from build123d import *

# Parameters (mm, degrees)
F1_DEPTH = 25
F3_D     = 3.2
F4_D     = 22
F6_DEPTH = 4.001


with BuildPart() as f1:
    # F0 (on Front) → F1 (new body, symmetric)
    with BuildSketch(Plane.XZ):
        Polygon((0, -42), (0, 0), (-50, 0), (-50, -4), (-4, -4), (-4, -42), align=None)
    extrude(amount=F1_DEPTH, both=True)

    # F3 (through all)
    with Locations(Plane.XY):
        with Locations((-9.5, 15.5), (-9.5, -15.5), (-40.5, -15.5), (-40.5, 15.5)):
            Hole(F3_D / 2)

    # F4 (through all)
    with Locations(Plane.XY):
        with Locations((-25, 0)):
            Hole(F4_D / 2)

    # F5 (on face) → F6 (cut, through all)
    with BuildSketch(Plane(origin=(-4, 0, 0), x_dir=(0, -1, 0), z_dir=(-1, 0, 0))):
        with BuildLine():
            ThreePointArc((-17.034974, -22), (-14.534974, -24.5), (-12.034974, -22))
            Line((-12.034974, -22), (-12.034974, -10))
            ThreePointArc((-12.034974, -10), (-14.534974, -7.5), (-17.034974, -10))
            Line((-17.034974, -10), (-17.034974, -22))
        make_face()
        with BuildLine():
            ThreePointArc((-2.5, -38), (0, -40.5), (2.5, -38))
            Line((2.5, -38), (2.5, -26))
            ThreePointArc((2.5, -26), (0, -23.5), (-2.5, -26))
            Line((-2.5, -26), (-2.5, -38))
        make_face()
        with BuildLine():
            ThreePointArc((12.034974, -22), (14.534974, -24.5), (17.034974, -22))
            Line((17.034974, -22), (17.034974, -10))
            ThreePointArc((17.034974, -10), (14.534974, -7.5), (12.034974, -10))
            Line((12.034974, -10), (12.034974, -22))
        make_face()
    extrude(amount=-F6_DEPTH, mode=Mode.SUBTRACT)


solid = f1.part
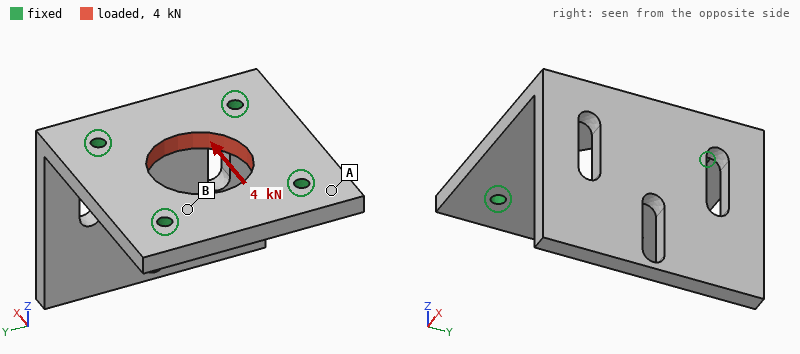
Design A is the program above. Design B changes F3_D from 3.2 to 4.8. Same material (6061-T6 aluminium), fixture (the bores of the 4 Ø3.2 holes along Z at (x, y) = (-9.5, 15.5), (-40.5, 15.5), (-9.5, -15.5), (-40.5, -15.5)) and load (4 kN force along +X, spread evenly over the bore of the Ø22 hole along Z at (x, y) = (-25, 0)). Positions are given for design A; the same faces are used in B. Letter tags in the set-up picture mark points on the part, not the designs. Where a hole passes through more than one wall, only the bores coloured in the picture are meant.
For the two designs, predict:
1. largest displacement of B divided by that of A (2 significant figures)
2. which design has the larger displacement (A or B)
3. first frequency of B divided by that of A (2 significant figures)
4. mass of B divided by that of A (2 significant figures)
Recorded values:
0.89
A
1.0
0.99
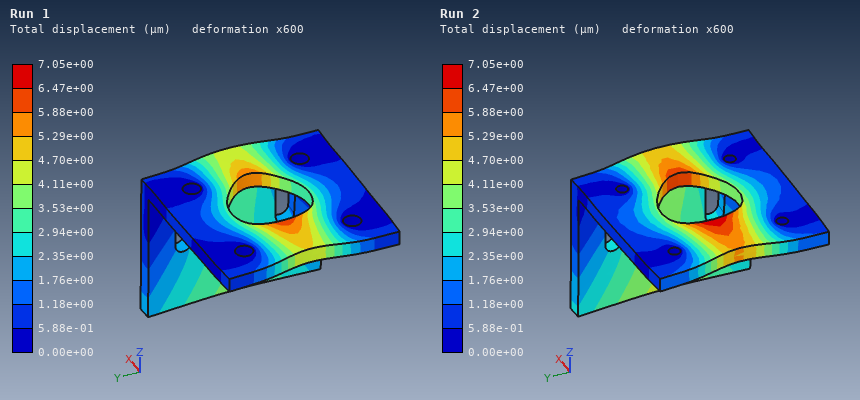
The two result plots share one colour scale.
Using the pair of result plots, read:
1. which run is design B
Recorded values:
Run 1
